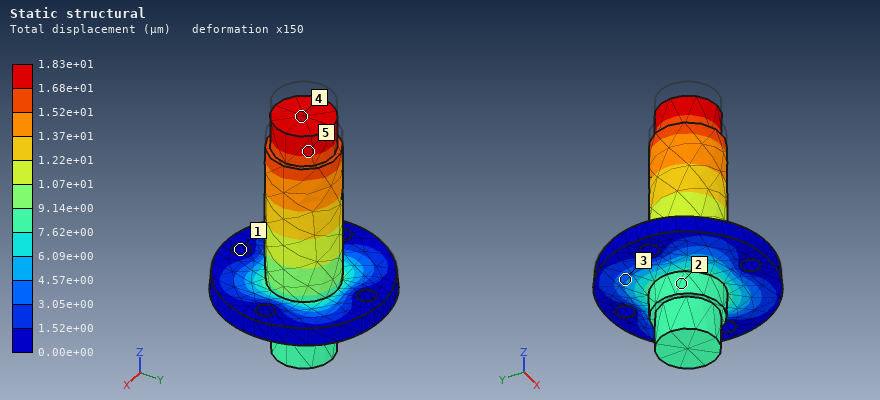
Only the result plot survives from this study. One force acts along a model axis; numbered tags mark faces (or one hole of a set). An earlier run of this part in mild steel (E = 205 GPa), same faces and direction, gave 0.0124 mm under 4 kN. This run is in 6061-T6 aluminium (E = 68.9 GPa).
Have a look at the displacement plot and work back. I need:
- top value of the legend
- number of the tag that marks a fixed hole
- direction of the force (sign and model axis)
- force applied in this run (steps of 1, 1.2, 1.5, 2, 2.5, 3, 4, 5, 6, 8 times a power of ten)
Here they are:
1.83e+01 µm
1
-Z
2 kN
